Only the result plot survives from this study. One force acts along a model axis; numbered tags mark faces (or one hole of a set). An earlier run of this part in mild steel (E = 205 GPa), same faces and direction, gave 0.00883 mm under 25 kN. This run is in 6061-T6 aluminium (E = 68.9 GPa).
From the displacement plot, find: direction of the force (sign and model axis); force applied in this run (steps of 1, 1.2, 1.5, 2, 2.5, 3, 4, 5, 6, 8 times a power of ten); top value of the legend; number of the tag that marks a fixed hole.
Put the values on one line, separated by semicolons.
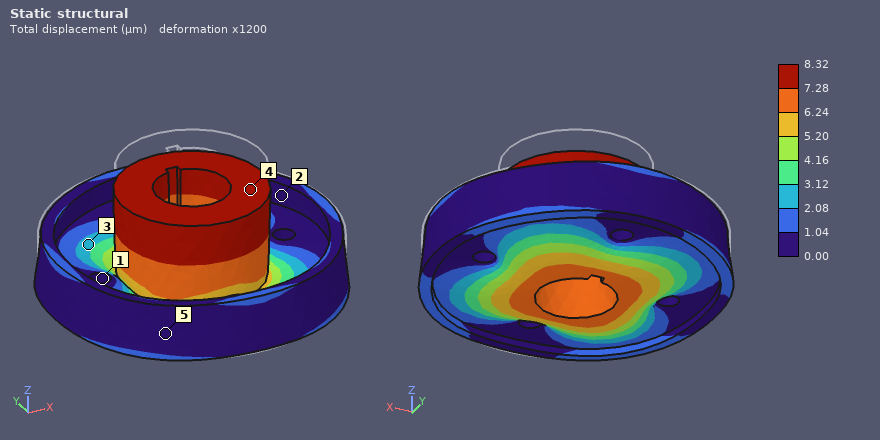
-Z; 8 kN; 8.32 µm; 1
